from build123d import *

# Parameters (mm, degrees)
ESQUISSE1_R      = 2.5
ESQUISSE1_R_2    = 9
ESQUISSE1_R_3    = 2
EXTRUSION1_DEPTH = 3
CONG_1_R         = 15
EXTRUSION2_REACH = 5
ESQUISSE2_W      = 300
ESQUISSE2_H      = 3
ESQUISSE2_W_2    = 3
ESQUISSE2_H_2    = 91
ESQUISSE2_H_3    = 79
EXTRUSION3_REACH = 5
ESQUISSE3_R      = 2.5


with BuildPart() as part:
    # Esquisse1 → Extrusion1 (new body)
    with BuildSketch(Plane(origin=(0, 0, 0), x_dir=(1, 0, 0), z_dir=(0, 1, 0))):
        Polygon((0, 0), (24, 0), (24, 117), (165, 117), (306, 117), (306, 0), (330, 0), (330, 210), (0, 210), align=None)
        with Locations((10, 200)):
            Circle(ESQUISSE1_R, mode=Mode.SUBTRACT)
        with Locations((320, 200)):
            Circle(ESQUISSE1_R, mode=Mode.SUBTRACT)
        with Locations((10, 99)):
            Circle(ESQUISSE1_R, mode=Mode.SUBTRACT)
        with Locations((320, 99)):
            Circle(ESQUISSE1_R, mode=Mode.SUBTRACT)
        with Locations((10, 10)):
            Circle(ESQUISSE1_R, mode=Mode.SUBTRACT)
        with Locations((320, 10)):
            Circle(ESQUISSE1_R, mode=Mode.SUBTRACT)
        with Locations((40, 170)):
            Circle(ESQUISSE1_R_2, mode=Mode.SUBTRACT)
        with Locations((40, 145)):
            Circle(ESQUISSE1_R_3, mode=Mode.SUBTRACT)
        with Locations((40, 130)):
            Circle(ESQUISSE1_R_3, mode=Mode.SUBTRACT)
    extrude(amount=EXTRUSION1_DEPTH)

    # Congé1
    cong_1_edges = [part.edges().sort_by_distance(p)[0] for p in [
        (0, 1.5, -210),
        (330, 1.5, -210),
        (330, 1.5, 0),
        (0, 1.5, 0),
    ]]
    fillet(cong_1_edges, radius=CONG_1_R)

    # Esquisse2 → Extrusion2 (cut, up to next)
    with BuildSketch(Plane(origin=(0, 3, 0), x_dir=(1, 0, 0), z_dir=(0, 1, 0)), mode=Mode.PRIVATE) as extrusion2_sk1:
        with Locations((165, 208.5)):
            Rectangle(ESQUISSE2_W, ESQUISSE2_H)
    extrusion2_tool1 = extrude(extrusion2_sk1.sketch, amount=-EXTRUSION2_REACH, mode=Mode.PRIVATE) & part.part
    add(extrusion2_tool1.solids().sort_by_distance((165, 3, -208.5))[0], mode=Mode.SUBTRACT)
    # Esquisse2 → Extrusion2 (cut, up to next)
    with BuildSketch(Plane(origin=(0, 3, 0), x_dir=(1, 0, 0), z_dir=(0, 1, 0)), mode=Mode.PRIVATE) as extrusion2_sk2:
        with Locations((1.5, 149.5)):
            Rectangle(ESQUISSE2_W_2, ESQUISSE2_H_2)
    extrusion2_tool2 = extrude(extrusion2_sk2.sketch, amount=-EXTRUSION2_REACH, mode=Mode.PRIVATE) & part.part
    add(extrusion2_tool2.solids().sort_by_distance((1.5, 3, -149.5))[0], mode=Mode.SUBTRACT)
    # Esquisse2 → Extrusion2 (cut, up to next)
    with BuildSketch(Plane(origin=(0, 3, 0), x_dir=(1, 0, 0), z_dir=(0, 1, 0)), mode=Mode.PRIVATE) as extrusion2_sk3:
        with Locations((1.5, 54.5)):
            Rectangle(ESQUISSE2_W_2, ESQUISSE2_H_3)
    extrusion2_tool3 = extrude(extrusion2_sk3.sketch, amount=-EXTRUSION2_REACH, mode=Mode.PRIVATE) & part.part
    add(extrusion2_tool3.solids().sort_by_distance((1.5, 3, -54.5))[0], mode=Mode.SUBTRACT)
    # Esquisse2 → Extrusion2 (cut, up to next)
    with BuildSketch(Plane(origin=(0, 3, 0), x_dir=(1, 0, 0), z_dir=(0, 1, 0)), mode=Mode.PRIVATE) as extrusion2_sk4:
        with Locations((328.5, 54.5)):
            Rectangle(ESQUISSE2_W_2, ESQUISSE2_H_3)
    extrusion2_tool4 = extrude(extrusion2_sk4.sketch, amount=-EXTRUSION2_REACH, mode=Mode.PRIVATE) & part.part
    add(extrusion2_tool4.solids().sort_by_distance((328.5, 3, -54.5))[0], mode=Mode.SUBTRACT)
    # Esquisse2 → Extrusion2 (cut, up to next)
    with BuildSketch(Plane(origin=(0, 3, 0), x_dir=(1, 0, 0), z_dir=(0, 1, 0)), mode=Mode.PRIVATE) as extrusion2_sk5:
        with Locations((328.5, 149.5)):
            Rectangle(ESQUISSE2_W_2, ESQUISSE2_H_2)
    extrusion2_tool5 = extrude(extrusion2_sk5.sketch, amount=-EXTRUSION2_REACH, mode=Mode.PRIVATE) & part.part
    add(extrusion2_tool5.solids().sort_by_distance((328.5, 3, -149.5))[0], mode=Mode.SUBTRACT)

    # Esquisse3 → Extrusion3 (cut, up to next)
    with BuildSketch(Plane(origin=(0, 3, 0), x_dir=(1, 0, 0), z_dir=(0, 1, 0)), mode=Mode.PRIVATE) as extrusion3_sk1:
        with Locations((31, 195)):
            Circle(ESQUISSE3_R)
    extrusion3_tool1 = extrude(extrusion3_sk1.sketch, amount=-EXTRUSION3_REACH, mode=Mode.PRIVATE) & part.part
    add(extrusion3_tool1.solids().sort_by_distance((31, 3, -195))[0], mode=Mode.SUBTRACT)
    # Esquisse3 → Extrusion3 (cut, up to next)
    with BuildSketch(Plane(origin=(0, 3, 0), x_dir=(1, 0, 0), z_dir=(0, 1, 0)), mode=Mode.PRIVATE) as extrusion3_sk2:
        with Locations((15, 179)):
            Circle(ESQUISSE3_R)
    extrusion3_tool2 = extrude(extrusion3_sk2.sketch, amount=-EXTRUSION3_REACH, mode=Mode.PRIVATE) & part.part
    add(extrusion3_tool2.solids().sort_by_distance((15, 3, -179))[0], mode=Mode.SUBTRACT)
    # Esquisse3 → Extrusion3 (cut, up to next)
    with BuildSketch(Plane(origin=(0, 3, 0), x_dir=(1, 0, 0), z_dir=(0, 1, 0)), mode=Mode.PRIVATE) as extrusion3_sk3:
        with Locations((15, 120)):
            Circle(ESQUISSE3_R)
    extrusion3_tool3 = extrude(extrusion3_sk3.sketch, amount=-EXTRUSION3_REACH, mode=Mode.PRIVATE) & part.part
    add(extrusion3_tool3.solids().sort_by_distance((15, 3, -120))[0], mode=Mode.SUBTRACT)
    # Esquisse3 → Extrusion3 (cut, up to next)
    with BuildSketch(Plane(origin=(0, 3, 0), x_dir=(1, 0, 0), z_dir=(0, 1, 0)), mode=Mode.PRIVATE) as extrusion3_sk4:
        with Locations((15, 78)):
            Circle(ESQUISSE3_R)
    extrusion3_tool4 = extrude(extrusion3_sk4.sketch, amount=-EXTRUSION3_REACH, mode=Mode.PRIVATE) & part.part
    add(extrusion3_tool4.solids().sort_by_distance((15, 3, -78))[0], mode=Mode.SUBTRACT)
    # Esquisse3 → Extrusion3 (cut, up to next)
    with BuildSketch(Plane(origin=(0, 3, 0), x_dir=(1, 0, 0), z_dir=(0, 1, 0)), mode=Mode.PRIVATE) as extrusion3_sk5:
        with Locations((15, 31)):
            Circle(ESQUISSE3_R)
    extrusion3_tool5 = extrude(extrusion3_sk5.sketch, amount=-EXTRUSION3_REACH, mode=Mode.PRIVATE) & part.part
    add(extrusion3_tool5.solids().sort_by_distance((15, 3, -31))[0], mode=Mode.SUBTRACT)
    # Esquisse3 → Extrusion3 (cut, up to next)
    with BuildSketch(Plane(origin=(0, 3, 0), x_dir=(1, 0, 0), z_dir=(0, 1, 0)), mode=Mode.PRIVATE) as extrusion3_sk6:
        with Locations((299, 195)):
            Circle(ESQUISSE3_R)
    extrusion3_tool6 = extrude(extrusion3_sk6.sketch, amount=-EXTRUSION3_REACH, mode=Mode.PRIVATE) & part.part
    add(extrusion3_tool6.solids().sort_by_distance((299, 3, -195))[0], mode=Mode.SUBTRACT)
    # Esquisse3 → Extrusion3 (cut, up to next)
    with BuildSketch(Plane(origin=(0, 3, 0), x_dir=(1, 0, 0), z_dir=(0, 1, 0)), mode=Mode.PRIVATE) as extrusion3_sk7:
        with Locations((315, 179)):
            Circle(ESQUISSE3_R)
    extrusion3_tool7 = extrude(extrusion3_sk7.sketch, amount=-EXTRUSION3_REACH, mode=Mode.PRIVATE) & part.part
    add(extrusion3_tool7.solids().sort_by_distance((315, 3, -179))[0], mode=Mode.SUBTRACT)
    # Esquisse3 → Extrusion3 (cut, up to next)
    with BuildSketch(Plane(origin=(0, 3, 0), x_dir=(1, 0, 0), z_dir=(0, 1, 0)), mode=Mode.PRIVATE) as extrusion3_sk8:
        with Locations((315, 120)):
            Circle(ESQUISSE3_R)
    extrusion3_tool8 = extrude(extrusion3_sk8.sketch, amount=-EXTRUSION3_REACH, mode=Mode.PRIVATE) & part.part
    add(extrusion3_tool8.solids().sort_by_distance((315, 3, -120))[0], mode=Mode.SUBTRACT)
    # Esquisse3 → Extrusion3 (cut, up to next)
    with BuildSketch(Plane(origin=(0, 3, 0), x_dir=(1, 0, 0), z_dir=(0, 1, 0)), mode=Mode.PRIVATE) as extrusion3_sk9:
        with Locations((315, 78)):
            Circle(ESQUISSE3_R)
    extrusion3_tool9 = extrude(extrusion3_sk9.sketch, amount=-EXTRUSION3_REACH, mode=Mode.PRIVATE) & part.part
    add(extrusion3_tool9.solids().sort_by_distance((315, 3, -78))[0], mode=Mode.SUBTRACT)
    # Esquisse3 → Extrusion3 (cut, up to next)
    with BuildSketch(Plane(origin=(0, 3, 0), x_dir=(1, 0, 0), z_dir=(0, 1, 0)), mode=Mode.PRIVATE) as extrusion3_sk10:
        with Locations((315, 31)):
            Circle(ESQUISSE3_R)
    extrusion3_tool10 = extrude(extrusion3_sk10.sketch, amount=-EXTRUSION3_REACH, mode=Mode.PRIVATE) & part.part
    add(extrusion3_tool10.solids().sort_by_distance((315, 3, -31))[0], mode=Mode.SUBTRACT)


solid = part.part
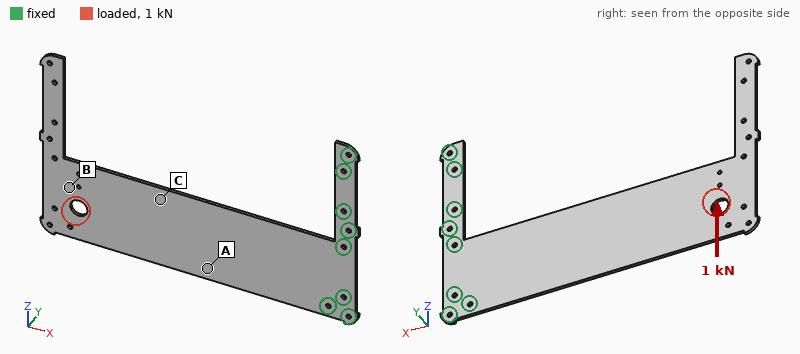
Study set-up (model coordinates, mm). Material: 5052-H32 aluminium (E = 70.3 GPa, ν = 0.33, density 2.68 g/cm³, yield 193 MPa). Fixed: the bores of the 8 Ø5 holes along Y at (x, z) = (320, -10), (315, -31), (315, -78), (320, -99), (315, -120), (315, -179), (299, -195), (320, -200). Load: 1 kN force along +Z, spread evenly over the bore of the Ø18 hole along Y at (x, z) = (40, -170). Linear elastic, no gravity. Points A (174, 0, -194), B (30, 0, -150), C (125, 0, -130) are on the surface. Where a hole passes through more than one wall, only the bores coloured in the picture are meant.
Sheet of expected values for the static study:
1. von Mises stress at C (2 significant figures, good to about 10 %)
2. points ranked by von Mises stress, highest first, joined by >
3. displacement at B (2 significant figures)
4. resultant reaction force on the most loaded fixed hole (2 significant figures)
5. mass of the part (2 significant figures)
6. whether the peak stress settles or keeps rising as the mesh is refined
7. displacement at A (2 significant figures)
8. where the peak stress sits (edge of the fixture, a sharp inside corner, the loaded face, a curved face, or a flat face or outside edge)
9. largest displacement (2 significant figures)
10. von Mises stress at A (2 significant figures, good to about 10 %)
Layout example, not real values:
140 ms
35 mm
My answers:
16 MPa
A > C > B
0.60 mm
3.3 kN
270 g
keeps rising
0.20 mm
edge of the fixture
0.83 mm
24 MPa
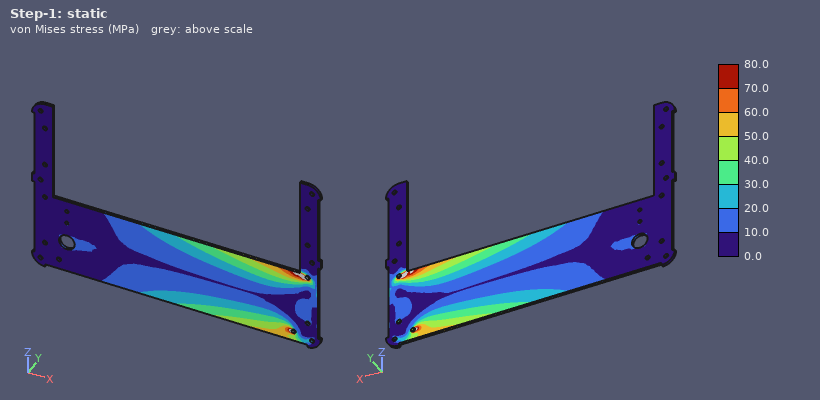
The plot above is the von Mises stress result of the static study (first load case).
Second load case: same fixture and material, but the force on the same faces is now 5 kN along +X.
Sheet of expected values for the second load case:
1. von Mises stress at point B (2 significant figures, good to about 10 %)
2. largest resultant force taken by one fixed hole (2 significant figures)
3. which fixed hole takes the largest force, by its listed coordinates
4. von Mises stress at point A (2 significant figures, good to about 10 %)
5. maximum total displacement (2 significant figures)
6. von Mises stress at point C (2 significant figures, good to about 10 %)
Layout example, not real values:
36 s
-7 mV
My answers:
12 MPa
1.8 kN
(299, -195)
26 MPa
0.14 mm
11 MPa
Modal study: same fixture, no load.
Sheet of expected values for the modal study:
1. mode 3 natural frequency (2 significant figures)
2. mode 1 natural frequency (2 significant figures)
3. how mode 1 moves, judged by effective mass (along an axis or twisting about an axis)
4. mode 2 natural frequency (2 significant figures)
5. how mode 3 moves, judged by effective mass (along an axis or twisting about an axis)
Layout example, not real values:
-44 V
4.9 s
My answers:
170 Hz
23 Hz
along Y
83 Hz
along Y
